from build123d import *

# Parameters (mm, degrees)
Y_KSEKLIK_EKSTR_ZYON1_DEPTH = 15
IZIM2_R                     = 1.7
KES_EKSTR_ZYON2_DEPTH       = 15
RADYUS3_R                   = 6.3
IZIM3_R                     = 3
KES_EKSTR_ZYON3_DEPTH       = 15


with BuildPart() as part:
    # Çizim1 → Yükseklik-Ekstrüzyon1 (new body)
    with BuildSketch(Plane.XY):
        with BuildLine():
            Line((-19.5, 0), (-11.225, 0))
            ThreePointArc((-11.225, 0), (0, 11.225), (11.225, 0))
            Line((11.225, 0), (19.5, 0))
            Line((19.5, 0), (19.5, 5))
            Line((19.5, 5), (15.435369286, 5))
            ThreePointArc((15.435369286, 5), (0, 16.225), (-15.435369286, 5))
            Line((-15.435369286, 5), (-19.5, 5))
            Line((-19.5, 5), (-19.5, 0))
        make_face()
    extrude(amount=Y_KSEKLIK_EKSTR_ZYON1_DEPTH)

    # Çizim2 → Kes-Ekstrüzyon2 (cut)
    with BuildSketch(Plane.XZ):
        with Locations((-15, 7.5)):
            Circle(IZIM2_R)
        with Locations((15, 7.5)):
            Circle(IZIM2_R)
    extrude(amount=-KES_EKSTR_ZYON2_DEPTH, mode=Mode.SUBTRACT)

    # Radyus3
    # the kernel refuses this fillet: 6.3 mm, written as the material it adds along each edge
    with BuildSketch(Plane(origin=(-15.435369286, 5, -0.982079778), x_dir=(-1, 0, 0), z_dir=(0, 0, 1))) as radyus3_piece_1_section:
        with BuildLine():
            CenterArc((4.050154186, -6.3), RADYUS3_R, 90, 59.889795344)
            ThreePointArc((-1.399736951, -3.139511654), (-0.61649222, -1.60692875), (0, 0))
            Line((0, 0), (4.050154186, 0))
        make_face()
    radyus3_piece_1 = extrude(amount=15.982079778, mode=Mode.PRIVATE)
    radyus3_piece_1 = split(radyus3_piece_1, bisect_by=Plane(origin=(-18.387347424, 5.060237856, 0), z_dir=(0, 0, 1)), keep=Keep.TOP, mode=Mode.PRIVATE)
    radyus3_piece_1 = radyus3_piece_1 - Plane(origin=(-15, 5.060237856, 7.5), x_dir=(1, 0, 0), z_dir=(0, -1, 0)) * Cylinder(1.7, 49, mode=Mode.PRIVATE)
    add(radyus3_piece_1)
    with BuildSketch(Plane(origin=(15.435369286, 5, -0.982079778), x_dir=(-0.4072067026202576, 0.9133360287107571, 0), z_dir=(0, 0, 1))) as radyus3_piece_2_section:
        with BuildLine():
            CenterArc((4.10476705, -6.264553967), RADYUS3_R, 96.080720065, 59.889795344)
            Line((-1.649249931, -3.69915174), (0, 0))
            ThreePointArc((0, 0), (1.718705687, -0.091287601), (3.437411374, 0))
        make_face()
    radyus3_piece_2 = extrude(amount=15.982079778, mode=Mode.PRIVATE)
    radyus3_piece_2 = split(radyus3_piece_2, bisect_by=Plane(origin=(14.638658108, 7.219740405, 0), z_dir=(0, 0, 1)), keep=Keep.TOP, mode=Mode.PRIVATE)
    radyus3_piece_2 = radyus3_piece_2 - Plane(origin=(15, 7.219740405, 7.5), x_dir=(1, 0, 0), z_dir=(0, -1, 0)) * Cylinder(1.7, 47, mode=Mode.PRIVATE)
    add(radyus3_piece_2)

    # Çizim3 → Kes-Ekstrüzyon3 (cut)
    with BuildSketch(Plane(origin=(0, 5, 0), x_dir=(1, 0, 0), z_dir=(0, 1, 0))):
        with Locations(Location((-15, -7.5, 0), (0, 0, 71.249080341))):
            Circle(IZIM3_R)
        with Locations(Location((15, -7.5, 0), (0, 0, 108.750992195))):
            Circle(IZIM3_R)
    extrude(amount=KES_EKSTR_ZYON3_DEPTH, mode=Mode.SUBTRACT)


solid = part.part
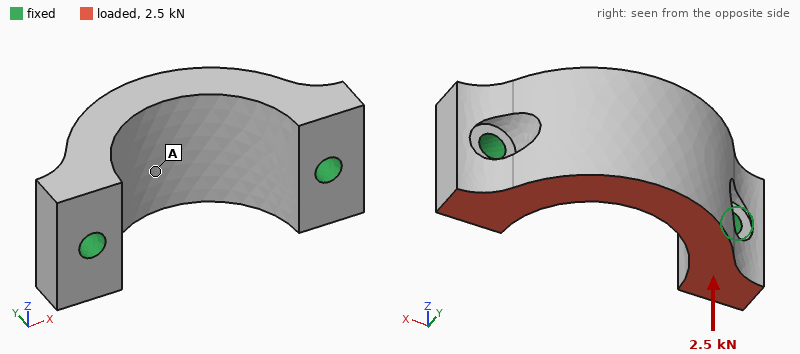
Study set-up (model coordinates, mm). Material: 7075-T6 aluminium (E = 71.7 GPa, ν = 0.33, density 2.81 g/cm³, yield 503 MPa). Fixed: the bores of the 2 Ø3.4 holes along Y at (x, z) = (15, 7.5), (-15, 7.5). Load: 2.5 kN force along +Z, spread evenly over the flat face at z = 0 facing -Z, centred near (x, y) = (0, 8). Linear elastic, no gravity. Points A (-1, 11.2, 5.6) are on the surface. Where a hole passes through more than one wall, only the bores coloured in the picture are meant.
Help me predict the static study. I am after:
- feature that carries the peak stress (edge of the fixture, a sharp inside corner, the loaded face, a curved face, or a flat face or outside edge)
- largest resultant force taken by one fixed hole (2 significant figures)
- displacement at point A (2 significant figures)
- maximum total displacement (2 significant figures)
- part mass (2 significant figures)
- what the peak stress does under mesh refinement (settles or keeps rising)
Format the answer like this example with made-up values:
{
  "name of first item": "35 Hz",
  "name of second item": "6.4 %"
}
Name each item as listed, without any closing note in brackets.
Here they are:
{
  "feature that carries the peak stress": "edge of the fixture",
  "largest resultant force taken by one fixed hole": "1.3 kN",
  "displacement at point A": "24 µm",
  "maximum total displacement": "40 µm",
  "part mass": "10 g",
  "what the peak stress does under mesh refinement": "keeps rising"
}
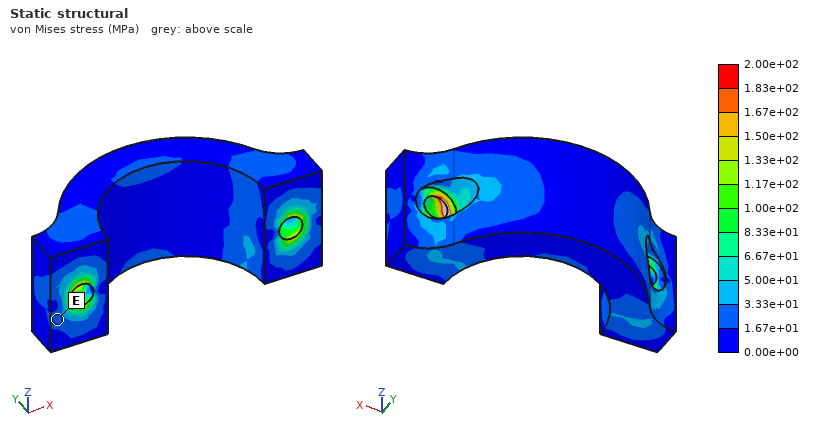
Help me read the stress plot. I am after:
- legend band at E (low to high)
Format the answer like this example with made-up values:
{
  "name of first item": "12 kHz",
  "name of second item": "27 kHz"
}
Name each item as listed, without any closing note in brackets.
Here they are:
{
  "legend band at E": "1.67e+01 to 3.33e+01 MPa"
}
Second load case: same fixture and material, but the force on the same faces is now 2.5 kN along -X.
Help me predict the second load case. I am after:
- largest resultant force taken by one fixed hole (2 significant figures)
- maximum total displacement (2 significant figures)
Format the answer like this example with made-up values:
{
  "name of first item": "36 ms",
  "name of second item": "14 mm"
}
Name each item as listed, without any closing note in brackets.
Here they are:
{
  "largest resultant force taken by one fixed hole": "1.4 kN",
  "maximum total displacement": "22 µm"
}
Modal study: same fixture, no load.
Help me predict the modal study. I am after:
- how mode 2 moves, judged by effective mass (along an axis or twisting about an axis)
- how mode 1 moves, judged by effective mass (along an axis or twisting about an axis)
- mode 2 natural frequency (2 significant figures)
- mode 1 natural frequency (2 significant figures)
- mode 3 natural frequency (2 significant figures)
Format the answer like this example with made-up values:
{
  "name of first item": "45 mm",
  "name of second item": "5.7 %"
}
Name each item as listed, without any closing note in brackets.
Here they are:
{
  "how mode 2 moves, judged by effective mass": "along X",
  "how mode 1 moves, judged by effective mass": "along Z",
  "mode 2 natural frequency": "26 kHz",
  "mode 1 natural frequency": "15 kHz",
  "mode 3 natural frequency": "32 kHz"
}
